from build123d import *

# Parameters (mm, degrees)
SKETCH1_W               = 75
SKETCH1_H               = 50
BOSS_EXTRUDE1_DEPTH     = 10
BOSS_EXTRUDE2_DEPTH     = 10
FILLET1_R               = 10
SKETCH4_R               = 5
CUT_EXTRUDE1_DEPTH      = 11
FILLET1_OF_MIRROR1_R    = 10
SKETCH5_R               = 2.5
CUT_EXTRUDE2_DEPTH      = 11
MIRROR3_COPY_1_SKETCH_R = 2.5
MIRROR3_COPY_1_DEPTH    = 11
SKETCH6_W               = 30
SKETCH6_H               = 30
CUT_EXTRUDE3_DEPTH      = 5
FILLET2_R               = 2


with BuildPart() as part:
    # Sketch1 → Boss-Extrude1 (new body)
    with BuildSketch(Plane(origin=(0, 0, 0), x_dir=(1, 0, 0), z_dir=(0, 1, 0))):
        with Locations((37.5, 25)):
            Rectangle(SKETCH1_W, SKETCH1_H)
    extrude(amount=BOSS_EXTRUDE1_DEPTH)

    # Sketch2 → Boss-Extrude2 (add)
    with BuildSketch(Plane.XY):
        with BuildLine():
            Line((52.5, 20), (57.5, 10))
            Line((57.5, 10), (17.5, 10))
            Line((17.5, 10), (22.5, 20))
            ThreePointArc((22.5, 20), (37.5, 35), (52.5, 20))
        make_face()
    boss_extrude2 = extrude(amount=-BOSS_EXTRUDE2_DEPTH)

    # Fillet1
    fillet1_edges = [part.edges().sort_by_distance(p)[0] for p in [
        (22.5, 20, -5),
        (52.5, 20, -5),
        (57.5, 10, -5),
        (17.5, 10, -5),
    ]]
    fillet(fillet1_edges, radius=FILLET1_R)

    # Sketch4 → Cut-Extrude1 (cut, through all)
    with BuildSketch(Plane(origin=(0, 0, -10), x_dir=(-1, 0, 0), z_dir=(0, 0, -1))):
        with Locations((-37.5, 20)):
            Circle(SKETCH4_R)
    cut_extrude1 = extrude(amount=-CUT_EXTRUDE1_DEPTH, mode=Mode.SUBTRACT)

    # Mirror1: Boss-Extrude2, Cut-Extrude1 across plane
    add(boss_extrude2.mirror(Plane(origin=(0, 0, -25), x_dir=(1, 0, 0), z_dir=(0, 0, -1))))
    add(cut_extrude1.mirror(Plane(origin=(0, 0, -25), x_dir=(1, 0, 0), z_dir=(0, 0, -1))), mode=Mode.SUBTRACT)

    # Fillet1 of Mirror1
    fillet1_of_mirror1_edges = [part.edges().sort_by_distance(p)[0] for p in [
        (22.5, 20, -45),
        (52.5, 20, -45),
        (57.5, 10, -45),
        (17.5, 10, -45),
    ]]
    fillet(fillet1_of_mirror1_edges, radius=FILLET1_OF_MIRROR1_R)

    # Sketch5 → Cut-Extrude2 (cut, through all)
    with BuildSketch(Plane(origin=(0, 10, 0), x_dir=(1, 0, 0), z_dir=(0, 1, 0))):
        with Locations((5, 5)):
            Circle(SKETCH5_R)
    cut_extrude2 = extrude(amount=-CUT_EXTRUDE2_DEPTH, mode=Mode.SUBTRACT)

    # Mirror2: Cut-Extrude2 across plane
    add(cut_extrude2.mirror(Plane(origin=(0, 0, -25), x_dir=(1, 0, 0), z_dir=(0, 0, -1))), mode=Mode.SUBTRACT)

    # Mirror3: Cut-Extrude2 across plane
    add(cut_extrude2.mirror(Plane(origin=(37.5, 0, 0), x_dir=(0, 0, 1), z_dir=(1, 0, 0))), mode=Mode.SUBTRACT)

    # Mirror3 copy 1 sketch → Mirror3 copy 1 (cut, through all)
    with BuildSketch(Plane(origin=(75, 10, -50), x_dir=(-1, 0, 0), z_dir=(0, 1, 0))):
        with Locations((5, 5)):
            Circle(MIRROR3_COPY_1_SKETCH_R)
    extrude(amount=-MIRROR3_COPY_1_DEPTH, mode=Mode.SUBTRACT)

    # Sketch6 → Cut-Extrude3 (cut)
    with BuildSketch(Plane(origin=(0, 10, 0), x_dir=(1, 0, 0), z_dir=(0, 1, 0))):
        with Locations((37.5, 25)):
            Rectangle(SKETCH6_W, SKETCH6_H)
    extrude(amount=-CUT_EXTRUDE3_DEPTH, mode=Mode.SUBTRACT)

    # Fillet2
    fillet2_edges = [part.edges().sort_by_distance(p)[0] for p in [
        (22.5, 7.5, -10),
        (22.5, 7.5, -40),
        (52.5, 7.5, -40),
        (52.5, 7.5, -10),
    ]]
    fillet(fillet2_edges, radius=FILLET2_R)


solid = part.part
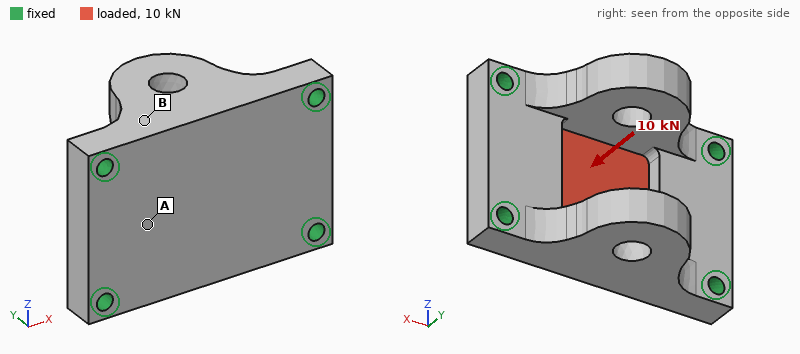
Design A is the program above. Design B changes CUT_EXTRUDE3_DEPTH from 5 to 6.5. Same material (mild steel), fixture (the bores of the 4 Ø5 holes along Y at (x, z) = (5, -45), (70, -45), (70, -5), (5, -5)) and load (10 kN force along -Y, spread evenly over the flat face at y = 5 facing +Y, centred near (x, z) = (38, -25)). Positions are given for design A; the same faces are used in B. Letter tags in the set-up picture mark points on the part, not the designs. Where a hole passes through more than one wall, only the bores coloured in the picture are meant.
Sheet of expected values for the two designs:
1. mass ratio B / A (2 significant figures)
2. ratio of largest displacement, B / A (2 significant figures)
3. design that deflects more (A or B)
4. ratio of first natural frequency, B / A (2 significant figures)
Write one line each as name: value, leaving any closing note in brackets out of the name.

mass ratio B / A: 0.97
ratio of largest displacement, B / A: 1.5
design that deflects more: B
ratio of first natural frequency, B / A: 0.98
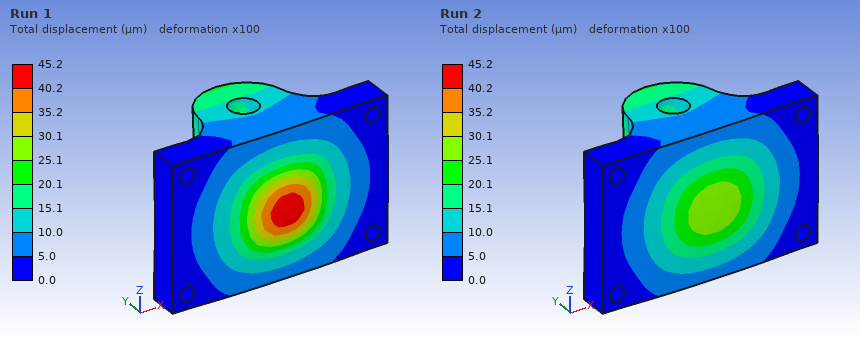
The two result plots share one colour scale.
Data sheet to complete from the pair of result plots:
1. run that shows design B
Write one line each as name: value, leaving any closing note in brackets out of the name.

run that shows design B: Run 1
